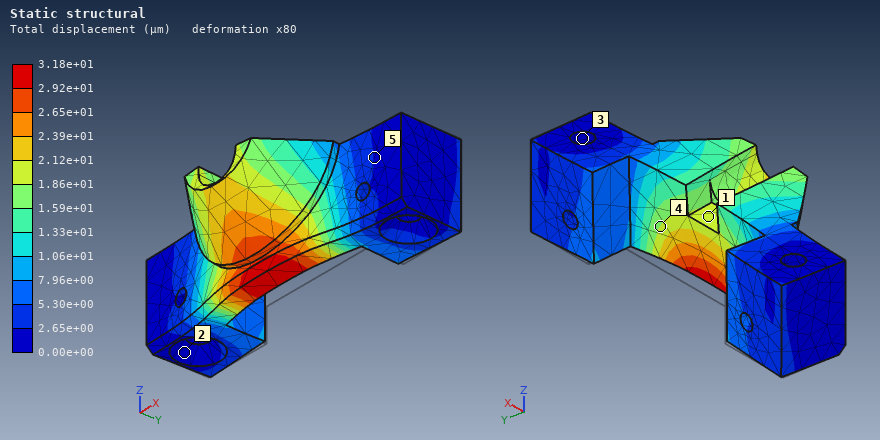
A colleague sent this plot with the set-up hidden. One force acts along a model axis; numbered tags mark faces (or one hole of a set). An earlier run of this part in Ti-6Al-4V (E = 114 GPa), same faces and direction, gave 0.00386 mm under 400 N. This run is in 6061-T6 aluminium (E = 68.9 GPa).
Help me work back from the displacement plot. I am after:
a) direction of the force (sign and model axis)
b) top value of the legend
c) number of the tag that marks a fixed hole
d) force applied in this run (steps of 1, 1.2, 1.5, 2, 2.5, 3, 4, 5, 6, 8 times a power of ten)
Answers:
-Y
3.18e+01 µm
3
2 kN
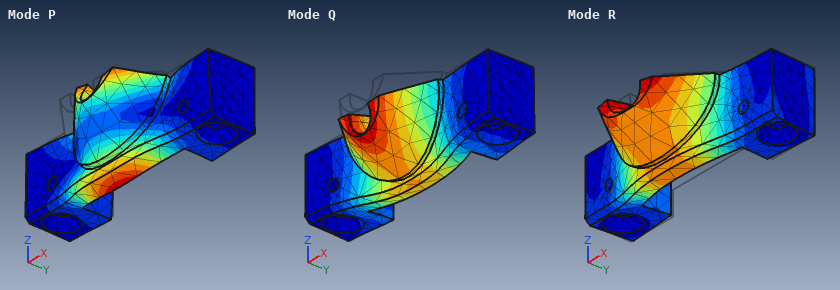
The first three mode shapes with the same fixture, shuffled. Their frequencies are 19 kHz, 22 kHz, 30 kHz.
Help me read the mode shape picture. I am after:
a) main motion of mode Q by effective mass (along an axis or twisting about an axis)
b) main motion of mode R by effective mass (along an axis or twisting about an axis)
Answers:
along Z
along Y
